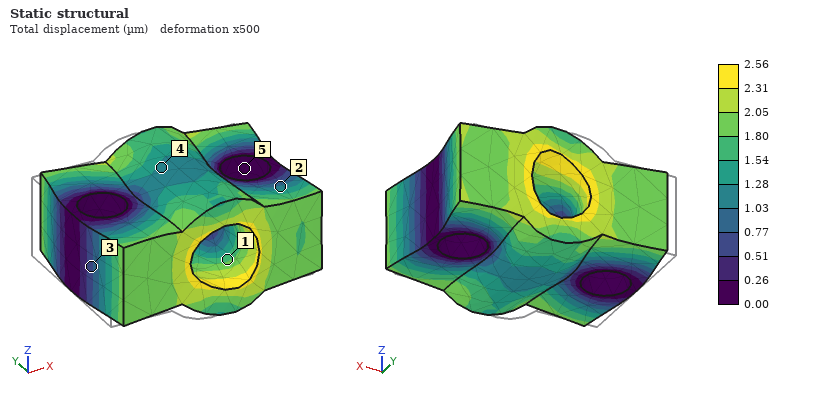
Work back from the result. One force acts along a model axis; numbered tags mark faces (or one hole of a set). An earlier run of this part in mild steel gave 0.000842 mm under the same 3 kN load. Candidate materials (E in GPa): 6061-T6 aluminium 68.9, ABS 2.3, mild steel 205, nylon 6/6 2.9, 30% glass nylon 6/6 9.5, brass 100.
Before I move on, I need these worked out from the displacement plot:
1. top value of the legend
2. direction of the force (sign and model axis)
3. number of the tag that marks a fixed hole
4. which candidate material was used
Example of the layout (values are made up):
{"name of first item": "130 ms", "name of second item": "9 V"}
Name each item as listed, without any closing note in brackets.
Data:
{"top value of the legend": "2.56 µm", "direction of the force": "+X", "number of the tag that marks a fixed hole": "5", "which candidate material was used": "6061-T6 aluminium"}
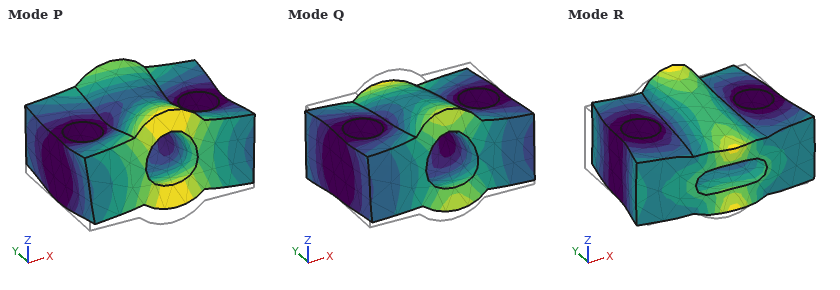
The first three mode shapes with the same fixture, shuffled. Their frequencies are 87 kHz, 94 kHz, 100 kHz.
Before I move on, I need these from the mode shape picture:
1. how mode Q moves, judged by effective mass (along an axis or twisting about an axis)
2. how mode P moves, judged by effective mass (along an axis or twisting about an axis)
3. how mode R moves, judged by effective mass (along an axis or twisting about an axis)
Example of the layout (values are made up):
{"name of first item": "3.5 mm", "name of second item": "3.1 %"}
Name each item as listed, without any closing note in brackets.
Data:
{"how mode Q moves, judged by effective mass": "twisting about X", "how mode P moves, judged by effective mass": "along Z", "how mode R moves, judged by effective mass": "along Y"}
